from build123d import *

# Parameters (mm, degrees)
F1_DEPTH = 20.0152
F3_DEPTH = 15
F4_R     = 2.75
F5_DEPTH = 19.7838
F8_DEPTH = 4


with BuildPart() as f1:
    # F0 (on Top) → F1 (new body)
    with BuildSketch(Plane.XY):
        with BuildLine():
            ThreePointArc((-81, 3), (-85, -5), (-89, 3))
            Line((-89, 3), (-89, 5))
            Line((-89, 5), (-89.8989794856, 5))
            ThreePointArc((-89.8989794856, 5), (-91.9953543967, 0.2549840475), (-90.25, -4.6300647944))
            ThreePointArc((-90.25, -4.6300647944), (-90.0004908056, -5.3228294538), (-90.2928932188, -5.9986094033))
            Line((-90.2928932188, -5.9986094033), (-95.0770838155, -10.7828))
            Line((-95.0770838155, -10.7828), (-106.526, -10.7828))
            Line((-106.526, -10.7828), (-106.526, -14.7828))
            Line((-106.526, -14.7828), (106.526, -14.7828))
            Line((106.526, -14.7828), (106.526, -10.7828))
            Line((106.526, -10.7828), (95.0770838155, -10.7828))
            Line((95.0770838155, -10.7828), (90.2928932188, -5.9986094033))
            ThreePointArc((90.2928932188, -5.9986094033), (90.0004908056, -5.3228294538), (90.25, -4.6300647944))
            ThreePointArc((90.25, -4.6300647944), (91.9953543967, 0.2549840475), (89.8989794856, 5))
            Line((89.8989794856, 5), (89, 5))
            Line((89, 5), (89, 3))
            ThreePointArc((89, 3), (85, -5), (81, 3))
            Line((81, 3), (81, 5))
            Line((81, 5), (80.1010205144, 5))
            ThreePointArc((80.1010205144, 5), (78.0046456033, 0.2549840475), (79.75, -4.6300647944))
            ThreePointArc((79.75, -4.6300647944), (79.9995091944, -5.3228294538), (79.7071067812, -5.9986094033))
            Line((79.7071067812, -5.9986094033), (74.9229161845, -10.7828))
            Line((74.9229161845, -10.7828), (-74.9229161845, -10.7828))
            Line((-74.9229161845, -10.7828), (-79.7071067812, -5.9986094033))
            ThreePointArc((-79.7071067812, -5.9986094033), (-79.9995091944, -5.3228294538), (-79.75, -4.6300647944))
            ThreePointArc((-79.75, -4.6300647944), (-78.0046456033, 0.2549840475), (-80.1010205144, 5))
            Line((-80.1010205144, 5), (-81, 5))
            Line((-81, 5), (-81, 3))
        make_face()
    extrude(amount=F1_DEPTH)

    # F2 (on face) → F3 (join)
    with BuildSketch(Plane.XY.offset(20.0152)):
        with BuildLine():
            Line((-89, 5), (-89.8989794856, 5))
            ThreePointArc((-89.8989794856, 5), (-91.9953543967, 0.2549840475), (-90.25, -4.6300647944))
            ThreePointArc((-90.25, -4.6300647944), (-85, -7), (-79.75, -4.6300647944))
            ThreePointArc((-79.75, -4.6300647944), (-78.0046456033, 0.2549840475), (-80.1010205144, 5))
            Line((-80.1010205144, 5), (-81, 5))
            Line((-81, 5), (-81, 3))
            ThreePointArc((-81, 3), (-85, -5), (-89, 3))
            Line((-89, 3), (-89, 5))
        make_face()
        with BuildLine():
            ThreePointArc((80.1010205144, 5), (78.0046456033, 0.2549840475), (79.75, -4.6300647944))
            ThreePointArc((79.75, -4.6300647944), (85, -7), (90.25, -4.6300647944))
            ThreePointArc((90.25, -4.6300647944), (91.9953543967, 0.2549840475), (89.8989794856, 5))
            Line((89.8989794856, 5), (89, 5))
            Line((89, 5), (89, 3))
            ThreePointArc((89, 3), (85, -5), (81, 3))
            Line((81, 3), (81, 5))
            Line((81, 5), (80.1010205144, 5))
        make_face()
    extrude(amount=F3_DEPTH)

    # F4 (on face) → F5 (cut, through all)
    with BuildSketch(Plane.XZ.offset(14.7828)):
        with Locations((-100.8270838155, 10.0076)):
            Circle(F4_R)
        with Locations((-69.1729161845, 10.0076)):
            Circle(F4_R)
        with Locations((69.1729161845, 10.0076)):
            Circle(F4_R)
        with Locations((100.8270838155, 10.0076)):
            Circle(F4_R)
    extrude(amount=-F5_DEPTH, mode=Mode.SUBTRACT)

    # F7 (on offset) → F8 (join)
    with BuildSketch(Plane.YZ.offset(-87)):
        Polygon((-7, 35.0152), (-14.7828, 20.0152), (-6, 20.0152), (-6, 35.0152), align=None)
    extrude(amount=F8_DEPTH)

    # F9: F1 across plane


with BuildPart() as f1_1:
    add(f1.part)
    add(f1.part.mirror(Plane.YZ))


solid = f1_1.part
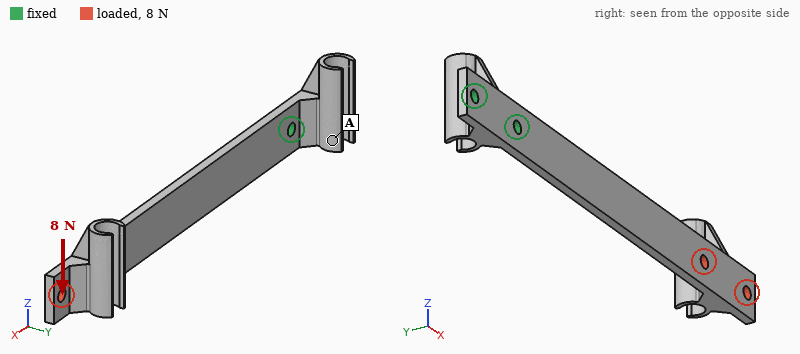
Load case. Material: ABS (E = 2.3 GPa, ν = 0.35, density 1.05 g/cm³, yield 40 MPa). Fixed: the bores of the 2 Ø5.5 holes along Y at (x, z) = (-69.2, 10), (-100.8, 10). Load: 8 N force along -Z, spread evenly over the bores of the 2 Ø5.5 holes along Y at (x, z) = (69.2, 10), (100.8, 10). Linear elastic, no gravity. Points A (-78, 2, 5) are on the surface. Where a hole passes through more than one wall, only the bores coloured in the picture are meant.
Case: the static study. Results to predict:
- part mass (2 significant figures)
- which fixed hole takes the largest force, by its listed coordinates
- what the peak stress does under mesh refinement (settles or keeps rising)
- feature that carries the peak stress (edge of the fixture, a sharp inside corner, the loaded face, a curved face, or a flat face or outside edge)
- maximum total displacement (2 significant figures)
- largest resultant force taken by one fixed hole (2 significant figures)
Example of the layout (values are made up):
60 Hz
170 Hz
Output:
25 g
(-69.2, 10)
keeps rising
edge of the fixture
2.2 mm
32 N
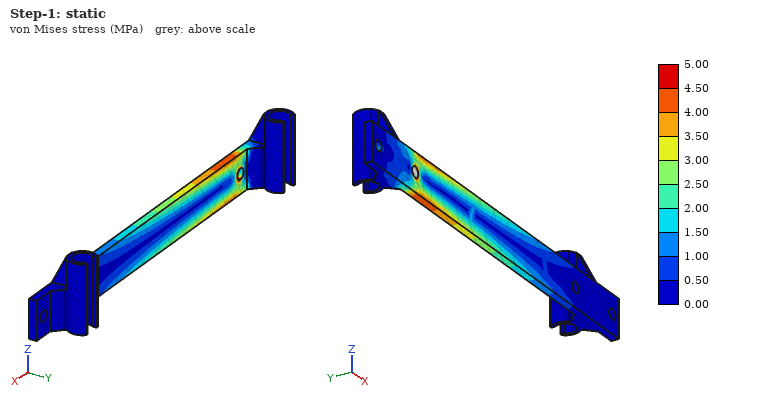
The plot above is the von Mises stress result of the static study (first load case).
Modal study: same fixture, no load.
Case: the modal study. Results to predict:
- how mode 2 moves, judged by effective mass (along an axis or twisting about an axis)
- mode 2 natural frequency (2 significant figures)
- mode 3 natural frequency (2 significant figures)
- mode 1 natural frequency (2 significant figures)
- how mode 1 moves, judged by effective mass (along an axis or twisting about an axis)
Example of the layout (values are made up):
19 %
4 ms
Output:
along Z
110 Hz
180 Hz
24 Hz
along Y
